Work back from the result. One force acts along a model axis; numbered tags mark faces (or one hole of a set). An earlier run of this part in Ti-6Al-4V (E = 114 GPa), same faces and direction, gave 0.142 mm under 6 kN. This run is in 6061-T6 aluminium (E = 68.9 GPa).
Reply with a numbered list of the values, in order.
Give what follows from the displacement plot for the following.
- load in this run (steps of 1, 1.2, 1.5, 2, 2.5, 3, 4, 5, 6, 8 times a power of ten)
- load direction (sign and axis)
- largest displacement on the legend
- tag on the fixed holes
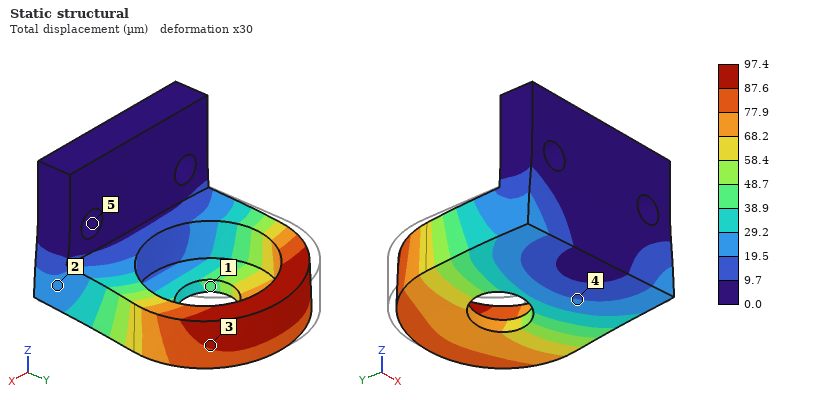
1. 2.5 kN
2. +X
3. 97.4 µm
4. 5
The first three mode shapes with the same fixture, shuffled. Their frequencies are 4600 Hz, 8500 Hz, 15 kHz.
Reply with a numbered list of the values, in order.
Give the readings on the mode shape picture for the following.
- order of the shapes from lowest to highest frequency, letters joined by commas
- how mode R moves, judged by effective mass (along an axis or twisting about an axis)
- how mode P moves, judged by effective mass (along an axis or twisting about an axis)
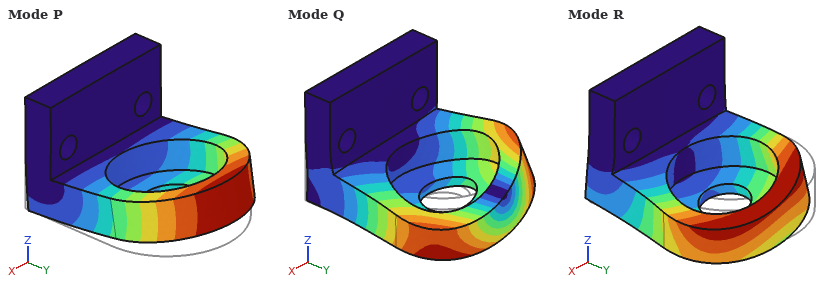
1. P, R, Q
2. along X
3. along Z
